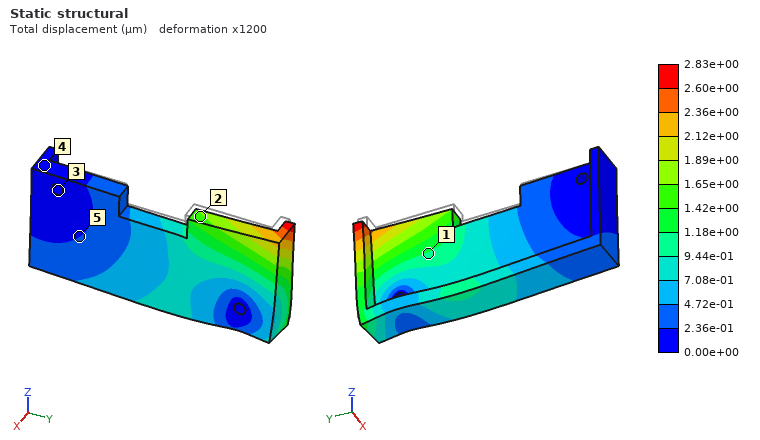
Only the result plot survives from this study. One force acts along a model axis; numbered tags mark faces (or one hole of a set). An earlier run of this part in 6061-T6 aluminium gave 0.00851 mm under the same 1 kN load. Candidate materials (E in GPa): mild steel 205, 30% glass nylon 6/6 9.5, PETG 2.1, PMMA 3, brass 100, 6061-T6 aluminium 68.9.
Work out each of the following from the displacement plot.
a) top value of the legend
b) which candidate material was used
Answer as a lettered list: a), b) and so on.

a) 2.83e+00 µm
b) mild steel
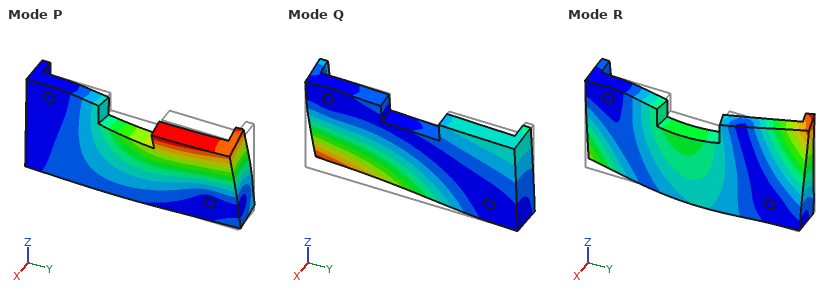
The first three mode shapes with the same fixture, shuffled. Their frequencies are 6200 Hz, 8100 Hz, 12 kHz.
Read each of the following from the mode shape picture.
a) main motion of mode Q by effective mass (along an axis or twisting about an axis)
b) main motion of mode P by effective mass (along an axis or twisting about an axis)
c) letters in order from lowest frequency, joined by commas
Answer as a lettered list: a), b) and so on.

a) along X
b) along X
c) Q, P, R
